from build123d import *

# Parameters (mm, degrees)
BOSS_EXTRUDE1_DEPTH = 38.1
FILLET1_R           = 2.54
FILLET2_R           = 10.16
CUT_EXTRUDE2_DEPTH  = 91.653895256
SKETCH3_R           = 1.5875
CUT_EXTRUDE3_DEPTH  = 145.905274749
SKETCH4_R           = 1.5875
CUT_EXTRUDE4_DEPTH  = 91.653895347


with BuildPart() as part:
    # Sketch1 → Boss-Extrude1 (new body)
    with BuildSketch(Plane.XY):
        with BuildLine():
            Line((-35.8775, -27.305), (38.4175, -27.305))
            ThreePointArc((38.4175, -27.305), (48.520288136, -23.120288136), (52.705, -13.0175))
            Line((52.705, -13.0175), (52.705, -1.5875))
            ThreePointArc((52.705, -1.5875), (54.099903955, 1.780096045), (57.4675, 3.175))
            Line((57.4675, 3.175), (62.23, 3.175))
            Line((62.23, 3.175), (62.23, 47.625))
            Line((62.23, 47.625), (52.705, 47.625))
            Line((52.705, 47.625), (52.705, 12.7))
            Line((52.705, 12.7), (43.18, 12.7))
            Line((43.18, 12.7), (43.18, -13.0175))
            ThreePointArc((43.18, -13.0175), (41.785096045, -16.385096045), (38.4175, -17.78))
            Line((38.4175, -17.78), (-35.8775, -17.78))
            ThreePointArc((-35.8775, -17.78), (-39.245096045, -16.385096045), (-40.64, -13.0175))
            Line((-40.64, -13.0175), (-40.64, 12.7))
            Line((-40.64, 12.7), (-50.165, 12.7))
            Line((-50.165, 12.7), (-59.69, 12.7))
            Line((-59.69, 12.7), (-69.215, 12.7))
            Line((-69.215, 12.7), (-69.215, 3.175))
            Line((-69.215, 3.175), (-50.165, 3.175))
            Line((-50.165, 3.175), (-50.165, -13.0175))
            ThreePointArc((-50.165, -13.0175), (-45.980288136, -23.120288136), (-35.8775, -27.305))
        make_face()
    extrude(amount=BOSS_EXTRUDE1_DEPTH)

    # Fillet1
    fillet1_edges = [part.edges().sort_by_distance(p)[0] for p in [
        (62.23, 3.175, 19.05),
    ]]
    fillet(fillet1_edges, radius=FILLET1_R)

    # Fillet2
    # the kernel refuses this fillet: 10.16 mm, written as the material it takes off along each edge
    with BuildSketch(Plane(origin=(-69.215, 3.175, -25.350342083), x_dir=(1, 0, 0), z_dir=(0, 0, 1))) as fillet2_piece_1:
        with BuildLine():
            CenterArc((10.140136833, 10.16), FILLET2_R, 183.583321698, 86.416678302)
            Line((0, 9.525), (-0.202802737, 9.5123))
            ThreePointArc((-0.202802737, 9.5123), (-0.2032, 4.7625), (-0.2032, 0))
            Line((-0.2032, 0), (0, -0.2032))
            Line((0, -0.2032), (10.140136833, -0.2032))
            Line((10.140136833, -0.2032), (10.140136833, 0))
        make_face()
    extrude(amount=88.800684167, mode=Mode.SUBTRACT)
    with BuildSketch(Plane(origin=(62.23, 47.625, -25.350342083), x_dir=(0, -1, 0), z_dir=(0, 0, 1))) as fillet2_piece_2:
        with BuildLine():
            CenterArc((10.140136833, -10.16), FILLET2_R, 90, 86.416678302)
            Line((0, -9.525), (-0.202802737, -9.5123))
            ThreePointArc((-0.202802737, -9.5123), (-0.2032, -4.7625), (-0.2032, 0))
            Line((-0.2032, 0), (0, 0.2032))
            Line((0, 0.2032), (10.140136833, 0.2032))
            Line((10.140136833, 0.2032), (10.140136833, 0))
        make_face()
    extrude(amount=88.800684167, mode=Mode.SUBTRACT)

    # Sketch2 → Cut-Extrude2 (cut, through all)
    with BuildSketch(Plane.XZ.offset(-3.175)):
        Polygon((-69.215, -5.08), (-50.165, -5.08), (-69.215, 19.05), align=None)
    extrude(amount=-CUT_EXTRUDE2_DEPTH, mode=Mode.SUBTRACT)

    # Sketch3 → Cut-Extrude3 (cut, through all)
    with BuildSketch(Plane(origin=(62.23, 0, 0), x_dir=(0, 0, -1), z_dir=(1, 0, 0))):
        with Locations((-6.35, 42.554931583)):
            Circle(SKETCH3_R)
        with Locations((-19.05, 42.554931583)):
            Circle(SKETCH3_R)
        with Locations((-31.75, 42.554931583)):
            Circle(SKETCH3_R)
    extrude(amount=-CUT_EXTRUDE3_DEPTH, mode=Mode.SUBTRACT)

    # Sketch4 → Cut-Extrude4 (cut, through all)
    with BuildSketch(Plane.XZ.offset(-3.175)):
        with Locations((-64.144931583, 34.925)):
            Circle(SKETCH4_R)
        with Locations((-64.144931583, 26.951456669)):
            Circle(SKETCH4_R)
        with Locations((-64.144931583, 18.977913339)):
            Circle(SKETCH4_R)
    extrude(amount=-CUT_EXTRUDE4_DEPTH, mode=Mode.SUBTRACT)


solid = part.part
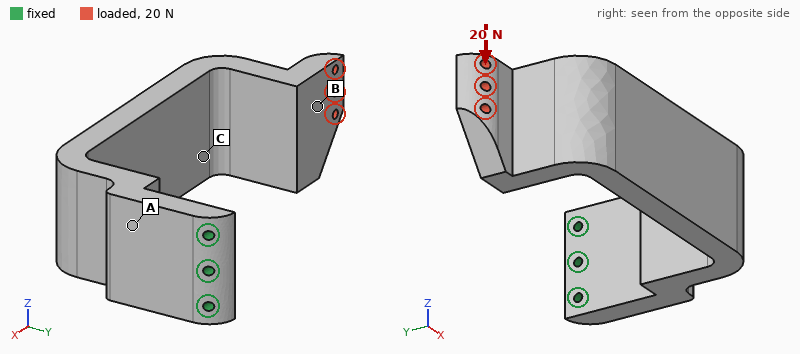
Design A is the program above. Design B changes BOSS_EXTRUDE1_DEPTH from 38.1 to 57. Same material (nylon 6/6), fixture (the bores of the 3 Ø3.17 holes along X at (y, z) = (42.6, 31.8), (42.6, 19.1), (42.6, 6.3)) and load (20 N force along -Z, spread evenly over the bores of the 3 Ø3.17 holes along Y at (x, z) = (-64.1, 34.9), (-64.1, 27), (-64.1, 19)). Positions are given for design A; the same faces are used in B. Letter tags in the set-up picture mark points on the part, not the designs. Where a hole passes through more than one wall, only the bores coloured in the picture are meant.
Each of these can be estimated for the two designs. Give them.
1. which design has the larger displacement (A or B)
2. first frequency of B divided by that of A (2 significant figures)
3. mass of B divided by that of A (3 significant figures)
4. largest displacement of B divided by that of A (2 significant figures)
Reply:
A
0.95
1.51
0.67
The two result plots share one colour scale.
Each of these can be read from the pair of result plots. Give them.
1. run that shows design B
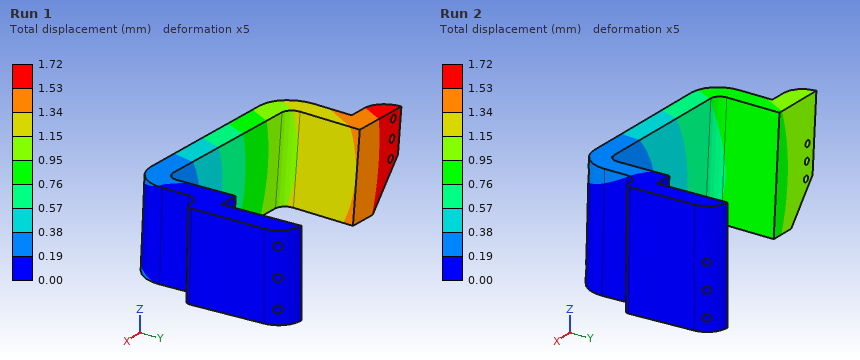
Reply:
Run 2
